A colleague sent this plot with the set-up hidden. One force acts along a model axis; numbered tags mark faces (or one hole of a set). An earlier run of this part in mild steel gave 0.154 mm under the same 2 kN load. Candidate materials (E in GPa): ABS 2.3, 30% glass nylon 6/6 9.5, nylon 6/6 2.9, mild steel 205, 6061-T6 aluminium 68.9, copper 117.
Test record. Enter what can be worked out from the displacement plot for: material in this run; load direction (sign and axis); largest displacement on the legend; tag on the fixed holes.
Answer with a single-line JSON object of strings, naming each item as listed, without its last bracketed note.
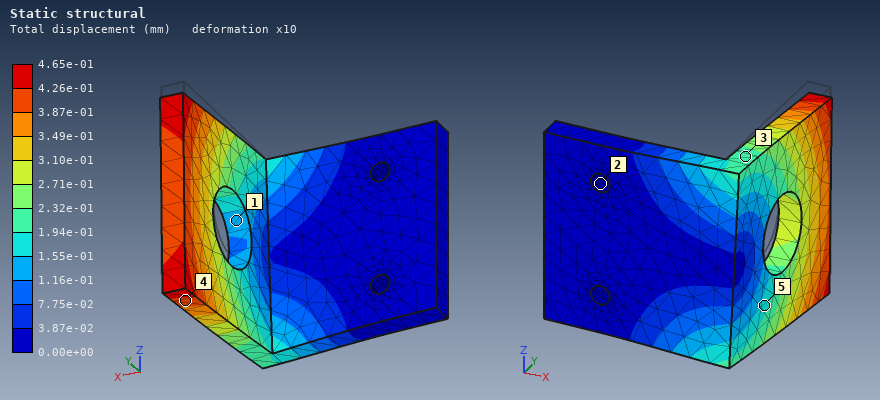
{"material in this run": "6061-T6 aluminium", "load direction": "-Z", "largest displacement on the legend": "4.65e-01 mm", "tag on the fixed holes": "2"}
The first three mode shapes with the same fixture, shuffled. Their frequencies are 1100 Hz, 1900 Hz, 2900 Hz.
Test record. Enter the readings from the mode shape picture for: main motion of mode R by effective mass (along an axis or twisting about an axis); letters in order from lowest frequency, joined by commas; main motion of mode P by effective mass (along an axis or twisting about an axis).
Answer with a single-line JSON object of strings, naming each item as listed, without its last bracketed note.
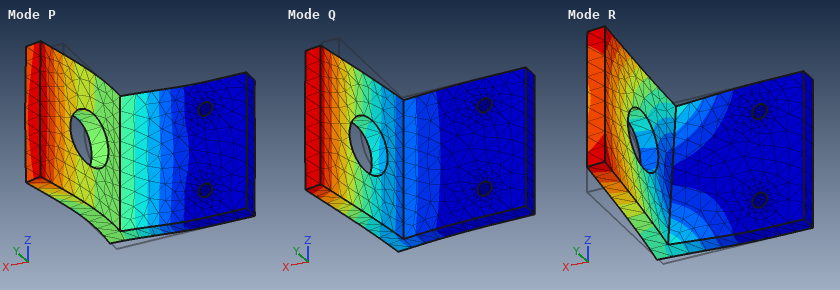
{"main motion of mode R by effective mass": "along Z", "letters in order from lowest frequency, joined by commas": "Q, R, P", "main motion of mode P by effective mass": "along Y"}
